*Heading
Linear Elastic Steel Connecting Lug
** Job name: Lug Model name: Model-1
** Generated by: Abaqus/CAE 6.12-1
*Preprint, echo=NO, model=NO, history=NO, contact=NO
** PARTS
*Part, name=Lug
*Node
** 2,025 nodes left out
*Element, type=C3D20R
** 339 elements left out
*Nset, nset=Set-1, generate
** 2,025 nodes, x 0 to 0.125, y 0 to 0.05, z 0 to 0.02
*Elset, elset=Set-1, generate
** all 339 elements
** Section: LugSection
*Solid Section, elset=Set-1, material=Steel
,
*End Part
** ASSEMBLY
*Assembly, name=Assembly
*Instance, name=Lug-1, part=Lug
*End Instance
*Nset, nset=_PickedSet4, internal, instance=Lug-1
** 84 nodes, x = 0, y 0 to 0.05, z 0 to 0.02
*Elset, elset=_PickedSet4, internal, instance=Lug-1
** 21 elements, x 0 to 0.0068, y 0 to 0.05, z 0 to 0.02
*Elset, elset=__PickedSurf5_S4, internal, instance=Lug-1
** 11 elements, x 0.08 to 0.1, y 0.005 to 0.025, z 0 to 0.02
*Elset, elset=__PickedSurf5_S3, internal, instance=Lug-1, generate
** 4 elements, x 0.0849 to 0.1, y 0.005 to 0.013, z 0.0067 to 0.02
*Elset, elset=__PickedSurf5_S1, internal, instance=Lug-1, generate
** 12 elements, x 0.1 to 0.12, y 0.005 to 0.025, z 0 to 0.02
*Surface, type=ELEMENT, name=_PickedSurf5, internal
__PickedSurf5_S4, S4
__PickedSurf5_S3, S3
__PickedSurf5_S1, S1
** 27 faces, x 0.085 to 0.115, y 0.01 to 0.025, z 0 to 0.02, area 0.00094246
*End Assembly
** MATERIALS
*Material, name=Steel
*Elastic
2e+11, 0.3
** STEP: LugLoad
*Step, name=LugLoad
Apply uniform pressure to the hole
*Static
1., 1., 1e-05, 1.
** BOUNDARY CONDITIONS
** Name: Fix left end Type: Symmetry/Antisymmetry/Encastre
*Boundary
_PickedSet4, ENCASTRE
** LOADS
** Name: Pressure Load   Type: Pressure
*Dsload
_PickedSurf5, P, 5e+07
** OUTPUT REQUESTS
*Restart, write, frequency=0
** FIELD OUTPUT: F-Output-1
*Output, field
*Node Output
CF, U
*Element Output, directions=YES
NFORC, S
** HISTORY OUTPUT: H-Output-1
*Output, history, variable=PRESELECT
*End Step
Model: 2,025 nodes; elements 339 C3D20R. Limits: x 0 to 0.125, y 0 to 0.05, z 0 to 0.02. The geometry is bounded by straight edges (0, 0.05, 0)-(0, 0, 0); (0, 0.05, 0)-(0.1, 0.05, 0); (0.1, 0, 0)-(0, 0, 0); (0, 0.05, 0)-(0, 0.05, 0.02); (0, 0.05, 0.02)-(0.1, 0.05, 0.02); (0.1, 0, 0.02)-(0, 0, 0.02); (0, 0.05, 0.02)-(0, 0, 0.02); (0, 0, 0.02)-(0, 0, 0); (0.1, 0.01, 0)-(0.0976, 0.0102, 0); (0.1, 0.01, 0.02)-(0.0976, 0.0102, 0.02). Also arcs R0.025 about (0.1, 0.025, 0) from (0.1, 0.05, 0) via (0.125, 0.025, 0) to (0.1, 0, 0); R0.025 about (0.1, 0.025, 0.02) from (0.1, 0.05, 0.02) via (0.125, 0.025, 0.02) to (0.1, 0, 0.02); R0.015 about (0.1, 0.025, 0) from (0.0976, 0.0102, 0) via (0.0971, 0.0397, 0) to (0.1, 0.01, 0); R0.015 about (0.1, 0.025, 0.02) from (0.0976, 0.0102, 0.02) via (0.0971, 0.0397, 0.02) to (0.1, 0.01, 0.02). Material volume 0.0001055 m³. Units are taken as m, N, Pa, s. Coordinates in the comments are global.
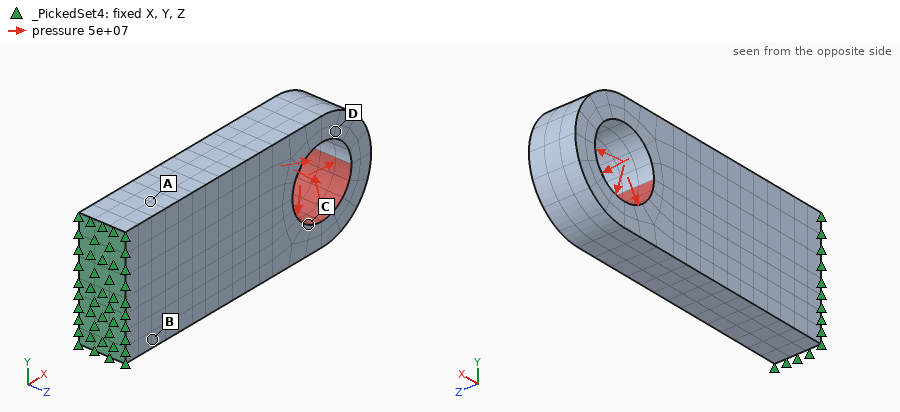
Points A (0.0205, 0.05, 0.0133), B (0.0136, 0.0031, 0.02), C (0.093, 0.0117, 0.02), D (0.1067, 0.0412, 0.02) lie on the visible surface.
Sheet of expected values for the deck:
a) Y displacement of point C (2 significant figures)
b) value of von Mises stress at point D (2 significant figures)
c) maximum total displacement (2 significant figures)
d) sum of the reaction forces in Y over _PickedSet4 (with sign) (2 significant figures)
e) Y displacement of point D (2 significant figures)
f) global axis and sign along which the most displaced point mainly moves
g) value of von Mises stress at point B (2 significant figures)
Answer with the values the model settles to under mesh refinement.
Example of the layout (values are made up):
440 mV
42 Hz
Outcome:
-2.7e-04 m
1.1e+08 Pa
4.2e-04 m
30000 N
-3.5e-04 m
-Y
2.7e+08 Pa
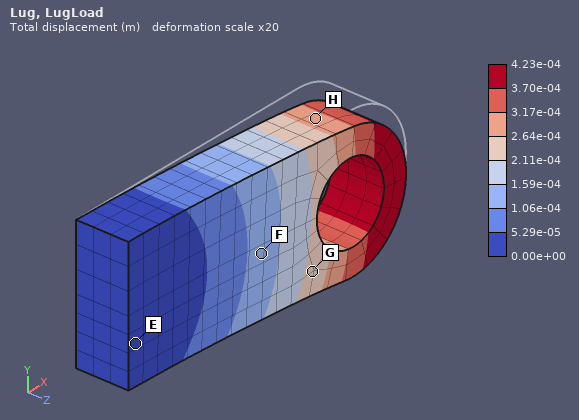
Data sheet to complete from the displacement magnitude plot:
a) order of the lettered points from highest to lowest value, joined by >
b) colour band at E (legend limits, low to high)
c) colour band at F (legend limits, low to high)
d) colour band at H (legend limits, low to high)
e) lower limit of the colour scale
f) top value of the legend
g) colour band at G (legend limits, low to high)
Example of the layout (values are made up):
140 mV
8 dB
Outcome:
H > G > F > E
0.00e+00 to 5.29e-05 m
1.06e-04 to 1.59e-04 m
2.64e-04 to 3.17e-04 m
0.00e+00 m
4.23e-04 m
2.11e-04 to 2.64e-04 m
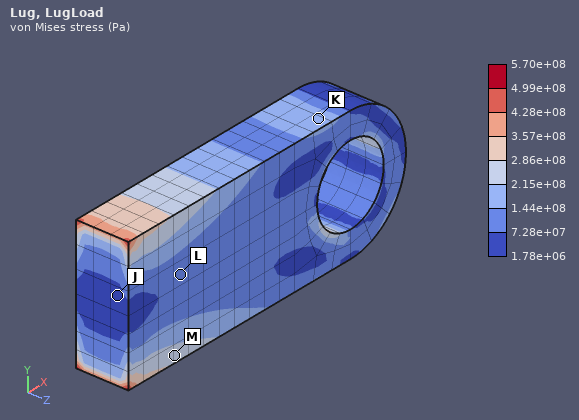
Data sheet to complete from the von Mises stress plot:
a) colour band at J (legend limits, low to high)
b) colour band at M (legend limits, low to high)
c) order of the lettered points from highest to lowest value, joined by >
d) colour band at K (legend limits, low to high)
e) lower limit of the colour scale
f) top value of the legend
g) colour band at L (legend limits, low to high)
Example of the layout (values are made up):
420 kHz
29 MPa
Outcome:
1.78e+06 to 7.28e+07 Pa
2.15e+08 to 2.86e+08 Pa
M > K > L > J
1.44e+08 to 2.15e+08 Pa
1.78e+06 Pa
5.70e+08 Pa
7.28e+07 to 1.44e+08 Pa
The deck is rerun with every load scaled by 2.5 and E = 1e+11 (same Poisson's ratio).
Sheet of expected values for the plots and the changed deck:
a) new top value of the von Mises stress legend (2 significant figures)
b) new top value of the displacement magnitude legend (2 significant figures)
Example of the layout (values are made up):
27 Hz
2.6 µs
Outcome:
1.4e+09 Pa
0.0021 m
